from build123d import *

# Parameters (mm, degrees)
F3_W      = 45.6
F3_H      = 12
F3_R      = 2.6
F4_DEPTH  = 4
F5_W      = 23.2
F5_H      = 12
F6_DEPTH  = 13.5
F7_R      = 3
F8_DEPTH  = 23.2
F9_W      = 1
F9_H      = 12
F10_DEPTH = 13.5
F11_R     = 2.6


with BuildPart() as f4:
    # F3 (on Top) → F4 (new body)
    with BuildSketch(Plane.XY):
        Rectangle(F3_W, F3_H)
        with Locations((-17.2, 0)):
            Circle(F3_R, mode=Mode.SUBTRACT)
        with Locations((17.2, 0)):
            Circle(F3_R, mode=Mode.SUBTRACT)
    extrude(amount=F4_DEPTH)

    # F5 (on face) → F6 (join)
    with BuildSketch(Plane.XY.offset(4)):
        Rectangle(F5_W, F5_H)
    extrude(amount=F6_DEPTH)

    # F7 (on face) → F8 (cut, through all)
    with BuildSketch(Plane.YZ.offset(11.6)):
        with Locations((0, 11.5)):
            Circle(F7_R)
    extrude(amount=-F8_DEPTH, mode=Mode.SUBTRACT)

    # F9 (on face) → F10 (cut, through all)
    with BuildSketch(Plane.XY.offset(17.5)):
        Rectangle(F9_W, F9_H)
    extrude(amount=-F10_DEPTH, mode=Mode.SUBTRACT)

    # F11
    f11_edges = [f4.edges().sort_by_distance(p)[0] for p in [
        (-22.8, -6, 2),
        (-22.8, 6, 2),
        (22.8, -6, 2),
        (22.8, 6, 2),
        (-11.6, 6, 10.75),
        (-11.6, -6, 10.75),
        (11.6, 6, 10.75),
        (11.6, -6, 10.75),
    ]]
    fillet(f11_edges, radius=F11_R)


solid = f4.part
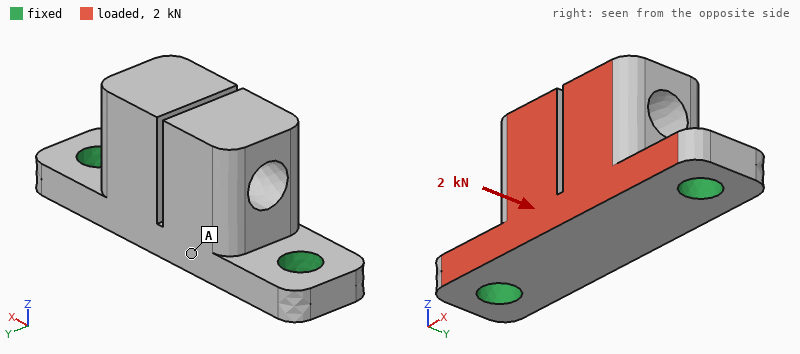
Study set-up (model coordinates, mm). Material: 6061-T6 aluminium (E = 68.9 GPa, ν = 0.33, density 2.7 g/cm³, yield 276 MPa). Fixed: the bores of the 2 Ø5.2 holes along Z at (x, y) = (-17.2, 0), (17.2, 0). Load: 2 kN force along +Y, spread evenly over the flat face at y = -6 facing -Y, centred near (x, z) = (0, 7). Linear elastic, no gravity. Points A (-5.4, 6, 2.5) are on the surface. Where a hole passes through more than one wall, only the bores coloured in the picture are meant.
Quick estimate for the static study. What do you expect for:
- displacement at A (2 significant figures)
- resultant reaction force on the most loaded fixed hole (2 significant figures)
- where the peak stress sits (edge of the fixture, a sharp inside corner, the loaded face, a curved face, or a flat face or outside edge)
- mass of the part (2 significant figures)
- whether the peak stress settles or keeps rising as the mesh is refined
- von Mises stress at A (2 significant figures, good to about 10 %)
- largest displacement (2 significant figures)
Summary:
26 µm
1.0 kN
edge of the fixture
13 g
keeps rising
25 MPa
82 µm
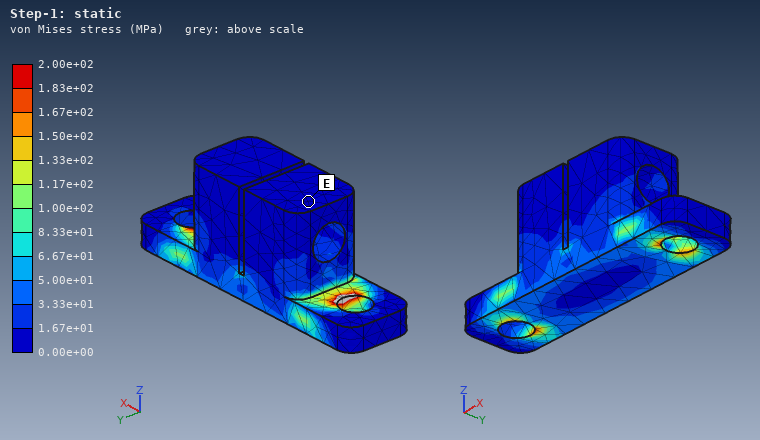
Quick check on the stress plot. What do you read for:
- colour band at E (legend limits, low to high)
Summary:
0.00e+00 to 1.67e+01 MPa
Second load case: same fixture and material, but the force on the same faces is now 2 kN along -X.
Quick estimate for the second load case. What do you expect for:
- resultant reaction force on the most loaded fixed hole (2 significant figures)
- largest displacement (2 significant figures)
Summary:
1.1 kN
16 µm
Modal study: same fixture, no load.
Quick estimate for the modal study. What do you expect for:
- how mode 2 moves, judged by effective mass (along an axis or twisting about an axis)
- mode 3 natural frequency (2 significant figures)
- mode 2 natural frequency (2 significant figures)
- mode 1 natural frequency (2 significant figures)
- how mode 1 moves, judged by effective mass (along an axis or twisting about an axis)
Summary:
along Z
16 kHz
9400 Hz
8200 Hz
along Y
